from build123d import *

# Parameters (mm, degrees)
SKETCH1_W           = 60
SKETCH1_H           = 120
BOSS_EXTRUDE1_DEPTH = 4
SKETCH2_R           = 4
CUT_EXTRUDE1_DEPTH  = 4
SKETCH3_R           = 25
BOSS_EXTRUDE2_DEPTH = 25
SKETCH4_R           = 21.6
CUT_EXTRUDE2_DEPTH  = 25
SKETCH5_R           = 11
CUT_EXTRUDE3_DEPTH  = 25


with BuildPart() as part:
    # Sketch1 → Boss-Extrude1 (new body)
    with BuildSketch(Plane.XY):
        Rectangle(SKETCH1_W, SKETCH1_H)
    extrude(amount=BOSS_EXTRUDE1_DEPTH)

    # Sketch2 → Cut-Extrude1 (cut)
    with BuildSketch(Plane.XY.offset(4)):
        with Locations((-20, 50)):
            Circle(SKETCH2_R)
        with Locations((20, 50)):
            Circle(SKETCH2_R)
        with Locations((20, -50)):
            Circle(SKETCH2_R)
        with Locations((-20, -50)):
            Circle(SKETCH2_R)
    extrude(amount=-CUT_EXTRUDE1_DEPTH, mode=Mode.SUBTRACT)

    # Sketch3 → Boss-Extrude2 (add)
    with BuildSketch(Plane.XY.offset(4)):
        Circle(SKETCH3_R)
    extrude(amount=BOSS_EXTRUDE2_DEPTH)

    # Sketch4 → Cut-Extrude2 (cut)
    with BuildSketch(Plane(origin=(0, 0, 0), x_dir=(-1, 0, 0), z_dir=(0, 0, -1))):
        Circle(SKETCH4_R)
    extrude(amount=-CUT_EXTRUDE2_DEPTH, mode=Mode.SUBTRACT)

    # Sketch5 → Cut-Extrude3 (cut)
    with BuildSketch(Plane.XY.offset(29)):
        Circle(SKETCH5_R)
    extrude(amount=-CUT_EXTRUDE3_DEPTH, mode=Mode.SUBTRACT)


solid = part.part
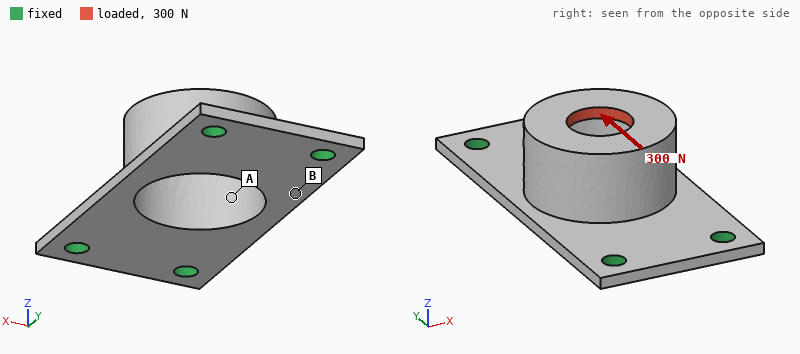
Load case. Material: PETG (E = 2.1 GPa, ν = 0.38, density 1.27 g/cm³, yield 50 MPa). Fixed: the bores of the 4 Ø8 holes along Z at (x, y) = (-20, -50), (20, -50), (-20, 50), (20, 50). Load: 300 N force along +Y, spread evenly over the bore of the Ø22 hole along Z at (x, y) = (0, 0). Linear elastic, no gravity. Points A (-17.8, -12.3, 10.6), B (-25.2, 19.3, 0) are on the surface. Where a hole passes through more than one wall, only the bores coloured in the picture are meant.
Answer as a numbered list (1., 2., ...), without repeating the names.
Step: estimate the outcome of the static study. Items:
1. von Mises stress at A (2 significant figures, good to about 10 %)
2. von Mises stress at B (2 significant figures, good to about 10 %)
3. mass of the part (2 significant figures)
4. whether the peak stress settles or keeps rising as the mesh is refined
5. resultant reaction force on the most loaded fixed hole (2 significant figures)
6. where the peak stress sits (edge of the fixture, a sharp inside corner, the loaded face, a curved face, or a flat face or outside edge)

1. 2.5 MPa
2. 4.8 MPa
3. 49 g
4. keeps rising
5. 93 N
6. edge of the fixture
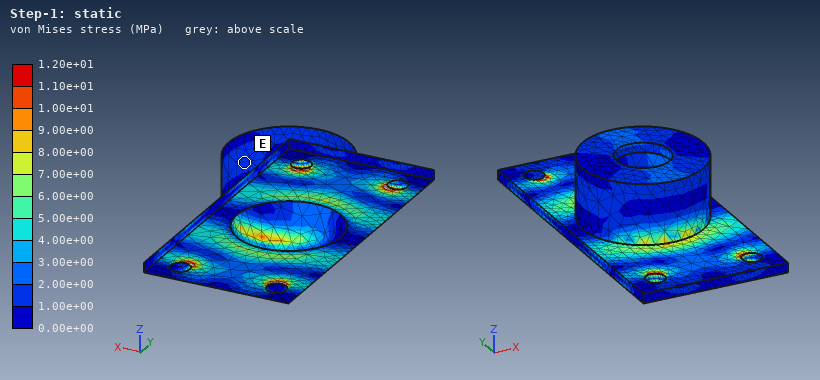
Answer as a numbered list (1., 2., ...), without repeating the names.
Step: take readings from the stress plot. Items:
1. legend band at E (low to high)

1. 1.00e+00 to 2.00e+00 MPa
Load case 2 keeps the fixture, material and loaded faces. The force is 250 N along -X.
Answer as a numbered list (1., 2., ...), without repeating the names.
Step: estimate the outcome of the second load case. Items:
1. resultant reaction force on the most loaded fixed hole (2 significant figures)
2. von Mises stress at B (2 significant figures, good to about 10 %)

1. 130 N
2. 8.2 MPa
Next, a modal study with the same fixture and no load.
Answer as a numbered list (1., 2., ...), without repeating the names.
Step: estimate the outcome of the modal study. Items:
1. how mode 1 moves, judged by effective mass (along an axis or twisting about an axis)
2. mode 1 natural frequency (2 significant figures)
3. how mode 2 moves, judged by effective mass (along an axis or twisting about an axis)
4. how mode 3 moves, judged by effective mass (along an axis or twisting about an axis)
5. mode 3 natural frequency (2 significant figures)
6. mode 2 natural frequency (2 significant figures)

1. along X
2. 510 Hz
3. along Z
4. along Y
5. 950 Hz
6. 620 Hz
